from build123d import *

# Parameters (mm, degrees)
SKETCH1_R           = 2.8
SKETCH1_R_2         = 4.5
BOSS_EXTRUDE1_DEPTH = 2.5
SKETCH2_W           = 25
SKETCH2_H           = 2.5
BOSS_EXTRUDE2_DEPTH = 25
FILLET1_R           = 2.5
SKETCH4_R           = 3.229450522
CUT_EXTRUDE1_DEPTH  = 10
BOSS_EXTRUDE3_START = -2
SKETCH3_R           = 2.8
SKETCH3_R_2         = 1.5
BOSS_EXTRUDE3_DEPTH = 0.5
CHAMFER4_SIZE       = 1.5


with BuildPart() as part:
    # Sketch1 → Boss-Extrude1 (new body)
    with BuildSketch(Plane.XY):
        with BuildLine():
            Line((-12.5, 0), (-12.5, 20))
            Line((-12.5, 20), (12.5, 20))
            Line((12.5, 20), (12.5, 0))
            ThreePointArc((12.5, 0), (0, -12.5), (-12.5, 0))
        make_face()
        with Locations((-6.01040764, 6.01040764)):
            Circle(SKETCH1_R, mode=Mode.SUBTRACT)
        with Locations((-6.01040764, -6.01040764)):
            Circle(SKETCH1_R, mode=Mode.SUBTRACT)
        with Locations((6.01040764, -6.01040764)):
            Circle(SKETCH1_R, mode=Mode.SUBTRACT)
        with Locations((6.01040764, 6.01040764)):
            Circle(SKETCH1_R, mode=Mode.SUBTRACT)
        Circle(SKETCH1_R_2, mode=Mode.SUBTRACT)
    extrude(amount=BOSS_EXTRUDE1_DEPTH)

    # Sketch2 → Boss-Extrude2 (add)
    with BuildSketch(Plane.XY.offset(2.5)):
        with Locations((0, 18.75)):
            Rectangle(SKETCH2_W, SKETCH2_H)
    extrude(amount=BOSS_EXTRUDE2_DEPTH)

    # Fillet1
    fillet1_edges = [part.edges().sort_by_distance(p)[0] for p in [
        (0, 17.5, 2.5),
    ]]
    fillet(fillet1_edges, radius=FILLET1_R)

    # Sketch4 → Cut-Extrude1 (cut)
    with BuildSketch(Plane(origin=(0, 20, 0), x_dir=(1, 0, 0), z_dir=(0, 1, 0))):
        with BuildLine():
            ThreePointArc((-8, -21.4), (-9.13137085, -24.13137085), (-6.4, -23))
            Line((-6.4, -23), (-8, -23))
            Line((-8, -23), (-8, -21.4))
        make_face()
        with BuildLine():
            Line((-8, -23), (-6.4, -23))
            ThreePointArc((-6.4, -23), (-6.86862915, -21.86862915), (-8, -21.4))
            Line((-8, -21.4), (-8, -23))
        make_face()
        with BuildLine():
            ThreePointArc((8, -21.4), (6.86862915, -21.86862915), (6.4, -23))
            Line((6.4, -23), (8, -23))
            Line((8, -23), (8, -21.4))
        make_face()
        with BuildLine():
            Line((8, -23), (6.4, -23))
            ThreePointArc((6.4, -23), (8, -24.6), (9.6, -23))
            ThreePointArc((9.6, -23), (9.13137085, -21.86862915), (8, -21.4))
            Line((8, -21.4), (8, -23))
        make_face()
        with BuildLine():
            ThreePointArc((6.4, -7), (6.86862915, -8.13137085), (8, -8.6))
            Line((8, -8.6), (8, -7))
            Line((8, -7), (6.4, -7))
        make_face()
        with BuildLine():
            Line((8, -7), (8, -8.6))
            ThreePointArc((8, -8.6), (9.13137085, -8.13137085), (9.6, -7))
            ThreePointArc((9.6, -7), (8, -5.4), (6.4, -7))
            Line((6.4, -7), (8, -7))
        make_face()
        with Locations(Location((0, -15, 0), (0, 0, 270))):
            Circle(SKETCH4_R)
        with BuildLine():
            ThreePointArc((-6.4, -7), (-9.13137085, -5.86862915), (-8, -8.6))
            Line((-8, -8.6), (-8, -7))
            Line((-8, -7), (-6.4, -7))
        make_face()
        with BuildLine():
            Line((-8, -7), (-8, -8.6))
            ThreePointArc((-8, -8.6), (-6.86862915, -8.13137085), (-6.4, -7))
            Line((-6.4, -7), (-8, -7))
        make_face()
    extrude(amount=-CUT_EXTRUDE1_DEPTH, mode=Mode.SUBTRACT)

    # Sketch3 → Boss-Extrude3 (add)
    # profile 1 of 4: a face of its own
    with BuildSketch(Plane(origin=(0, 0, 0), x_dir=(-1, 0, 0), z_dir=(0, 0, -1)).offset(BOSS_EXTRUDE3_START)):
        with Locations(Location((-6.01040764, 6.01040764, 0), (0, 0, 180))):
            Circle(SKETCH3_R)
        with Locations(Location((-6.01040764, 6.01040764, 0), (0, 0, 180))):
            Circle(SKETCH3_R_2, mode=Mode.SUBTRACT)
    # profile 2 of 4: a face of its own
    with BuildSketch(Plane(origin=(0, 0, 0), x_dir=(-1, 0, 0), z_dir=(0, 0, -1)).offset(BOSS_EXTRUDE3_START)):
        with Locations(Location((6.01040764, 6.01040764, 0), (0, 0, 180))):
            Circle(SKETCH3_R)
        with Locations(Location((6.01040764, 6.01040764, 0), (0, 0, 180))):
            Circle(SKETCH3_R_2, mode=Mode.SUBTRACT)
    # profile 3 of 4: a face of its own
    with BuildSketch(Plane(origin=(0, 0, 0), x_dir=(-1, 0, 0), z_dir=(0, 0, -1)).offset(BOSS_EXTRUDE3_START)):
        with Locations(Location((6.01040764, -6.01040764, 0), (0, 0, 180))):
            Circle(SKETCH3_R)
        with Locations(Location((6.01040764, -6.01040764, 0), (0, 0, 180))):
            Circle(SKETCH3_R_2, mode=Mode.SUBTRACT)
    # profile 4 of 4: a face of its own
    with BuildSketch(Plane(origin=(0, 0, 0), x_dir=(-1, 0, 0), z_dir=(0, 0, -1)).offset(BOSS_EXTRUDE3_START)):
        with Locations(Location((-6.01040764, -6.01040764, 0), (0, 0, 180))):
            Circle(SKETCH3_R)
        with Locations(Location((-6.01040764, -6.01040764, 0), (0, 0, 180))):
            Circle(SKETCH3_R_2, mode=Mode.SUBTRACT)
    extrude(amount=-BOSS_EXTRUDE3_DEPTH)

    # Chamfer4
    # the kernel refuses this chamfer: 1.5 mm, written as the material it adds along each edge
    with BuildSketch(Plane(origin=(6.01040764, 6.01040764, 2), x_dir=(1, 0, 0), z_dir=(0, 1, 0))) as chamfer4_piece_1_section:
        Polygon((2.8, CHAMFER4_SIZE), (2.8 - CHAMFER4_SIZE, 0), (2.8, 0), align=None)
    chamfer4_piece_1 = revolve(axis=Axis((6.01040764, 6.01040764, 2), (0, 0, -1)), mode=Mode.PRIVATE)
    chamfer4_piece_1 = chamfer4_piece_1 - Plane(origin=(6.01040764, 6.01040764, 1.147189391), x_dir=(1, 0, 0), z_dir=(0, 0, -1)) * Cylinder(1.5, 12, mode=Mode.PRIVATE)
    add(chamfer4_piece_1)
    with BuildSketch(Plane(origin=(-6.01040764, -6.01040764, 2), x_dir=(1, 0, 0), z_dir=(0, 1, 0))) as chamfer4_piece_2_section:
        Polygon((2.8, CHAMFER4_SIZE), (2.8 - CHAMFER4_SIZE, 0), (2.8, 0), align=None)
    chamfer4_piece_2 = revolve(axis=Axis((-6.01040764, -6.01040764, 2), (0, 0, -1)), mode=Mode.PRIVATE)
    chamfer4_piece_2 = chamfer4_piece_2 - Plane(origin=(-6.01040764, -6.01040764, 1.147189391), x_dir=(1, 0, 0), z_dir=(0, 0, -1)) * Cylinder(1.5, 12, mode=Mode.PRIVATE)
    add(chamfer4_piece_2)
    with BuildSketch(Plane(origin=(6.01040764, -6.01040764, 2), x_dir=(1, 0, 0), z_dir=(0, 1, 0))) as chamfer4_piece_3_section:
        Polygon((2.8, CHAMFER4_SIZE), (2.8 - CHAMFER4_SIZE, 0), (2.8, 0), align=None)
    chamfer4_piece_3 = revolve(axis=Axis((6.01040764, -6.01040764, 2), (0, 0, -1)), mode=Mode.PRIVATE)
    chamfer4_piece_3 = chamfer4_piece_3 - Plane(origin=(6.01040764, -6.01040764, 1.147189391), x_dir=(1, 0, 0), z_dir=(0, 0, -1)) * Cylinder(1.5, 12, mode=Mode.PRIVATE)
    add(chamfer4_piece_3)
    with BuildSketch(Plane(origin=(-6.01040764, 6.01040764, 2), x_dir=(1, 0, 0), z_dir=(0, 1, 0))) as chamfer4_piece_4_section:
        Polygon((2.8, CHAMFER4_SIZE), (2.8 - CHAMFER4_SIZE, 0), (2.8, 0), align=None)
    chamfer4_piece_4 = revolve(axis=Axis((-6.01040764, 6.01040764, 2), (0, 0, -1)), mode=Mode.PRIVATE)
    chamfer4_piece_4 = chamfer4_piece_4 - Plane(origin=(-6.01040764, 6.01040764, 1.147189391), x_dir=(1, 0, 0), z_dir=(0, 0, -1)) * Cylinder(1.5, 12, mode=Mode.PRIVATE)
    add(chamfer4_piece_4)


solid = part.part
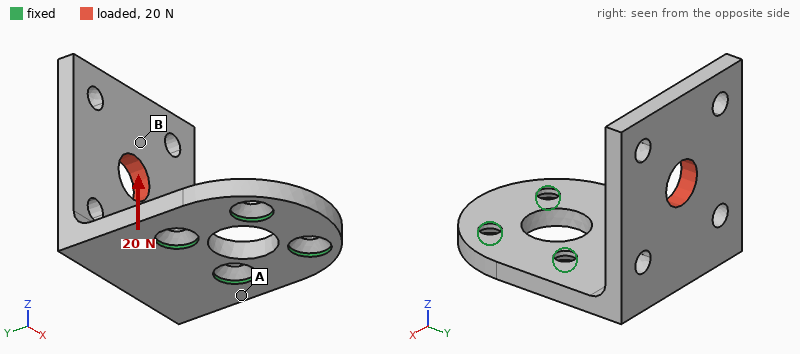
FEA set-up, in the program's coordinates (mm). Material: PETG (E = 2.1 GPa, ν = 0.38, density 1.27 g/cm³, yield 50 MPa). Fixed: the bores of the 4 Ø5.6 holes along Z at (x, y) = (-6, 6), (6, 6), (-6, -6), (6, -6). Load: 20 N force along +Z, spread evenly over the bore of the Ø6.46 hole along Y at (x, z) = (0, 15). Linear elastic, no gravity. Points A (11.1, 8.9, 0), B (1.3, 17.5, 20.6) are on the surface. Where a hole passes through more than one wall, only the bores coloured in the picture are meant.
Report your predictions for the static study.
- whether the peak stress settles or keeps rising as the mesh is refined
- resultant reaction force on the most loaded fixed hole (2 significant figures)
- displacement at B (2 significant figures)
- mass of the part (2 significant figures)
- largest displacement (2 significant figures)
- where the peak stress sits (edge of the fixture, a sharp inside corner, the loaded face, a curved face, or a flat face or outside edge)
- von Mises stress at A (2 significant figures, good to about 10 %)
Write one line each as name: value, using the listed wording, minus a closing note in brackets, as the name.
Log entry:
whether the peak stress settles or keeps rising as the mesh is refined: keeps rising
resultant reaction force on the most loaded fixed hole: 15 N
displacement at B: 0.42 mm
mass of the part: 3.8 g
largest displacement: 0.57 mm
where the peak stress sits: edge of the fixture
von Mises stress at A: 5.0 MPa
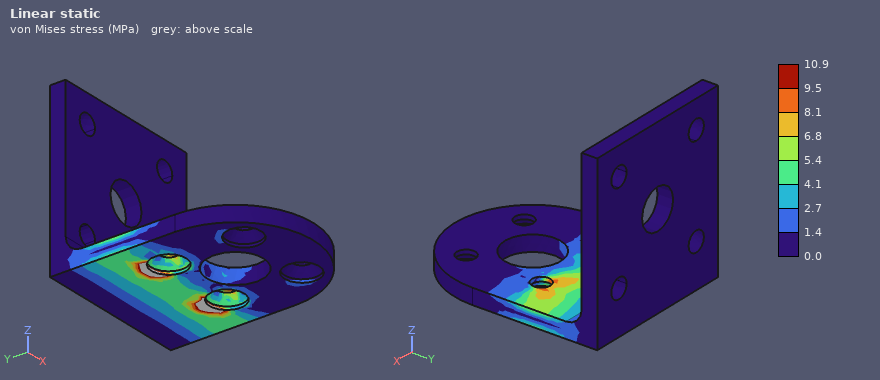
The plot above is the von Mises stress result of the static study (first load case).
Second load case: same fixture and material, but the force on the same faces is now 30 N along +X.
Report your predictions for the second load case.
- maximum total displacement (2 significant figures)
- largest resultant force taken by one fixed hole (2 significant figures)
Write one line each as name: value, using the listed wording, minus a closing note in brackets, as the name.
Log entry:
maximum total displacement: 0.57 mm
largest resultant force taken by one fixed hole: 49 N
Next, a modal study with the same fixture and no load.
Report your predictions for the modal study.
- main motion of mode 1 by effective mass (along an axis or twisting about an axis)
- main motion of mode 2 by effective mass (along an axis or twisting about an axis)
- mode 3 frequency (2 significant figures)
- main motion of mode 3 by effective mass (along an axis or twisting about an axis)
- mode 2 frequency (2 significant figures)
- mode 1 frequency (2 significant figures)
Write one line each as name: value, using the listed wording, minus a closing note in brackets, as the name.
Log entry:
main motion of mode 1 by effective mass: along Y
main motion of mode 2 by effective mass: along X
mode 3 frequency: 1700 Hz
main motion of mode 3 by effective mass: along Z
mode 2 frequency: 970 Hz
mode 1 frequency: 480 Hz
